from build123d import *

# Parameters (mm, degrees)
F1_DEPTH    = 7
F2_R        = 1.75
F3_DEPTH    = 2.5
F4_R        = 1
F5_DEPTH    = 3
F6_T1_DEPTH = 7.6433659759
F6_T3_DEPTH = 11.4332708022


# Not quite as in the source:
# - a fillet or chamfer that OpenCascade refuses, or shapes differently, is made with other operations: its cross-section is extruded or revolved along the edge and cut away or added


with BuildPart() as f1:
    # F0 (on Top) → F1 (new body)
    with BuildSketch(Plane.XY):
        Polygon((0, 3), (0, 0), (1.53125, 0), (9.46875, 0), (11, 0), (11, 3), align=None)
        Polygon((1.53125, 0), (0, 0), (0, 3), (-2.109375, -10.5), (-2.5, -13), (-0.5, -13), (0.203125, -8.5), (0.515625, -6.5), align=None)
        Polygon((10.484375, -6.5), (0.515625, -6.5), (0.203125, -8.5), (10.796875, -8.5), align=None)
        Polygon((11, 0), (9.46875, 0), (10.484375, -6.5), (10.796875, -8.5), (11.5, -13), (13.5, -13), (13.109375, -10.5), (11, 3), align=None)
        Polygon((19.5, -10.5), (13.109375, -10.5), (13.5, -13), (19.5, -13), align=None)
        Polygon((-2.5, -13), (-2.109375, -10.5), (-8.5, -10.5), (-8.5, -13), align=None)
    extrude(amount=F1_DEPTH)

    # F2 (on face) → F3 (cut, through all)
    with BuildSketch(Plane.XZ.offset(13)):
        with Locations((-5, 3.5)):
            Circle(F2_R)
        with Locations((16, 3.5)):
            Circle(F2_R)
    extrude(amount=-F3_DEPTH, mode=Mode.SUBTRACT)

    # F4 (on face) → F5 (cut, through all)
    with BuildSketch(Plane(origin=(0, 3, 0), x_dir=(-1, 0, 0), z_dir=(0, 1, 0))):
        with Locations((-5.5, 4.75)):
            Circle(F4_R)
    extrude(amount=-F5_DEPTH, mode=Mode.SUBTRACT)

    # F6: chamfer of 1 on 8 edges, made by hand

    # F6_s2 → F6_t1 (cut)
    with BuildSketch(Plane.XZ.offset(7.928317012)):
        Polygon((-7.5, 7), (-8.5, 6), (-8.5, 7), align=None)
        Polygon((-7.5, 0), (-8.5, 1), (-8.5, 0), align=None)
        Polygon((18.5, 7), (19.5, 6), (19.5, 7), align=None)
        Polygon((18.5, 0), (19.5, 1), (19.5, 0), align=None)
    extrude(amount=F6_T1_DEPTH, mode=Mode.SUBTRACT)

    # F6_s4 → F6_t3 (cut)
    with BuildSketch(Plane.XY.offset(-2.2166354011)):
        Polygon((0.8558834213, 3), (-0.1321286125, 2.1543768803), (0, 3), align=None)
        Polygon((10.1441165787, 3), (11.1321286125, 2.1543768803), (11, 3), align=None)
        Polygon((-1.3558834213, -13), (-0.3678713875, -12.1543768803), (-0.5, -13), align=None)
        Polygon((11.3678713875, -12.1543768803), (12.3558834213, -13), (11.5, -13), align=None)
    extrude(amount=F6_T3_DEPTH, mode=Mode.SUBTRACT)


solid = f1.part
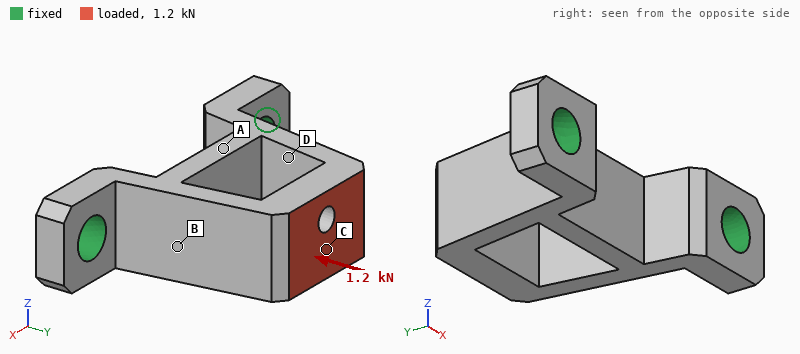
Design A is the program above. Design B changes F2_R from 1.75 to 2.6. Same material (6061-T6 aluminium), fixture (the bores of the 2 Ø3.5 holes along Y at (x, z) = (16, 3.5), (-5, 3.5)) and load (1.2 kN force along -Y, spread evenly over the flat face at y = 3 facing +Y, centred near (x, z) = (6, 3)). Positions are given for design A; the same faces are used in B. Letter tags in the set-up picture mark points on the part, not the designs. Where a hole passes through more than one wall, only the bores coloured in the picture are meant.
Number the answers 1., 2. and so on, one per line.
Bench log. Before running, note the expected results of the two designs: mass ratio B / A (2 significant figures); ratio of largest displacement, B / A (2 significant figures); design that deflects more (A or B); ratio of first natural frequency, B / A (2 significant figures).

1. 0.93
2. 0.86
3. A
4. 1.2
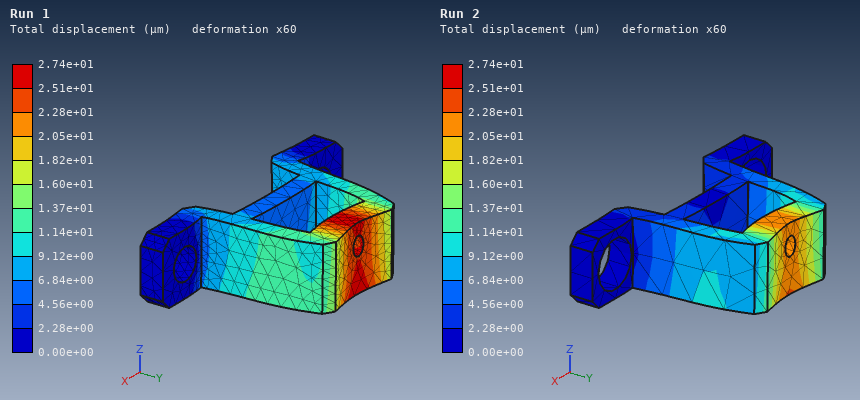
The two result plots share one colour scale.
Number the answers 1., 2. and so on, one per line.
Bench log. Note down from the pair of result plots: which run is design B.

1. Run 2
